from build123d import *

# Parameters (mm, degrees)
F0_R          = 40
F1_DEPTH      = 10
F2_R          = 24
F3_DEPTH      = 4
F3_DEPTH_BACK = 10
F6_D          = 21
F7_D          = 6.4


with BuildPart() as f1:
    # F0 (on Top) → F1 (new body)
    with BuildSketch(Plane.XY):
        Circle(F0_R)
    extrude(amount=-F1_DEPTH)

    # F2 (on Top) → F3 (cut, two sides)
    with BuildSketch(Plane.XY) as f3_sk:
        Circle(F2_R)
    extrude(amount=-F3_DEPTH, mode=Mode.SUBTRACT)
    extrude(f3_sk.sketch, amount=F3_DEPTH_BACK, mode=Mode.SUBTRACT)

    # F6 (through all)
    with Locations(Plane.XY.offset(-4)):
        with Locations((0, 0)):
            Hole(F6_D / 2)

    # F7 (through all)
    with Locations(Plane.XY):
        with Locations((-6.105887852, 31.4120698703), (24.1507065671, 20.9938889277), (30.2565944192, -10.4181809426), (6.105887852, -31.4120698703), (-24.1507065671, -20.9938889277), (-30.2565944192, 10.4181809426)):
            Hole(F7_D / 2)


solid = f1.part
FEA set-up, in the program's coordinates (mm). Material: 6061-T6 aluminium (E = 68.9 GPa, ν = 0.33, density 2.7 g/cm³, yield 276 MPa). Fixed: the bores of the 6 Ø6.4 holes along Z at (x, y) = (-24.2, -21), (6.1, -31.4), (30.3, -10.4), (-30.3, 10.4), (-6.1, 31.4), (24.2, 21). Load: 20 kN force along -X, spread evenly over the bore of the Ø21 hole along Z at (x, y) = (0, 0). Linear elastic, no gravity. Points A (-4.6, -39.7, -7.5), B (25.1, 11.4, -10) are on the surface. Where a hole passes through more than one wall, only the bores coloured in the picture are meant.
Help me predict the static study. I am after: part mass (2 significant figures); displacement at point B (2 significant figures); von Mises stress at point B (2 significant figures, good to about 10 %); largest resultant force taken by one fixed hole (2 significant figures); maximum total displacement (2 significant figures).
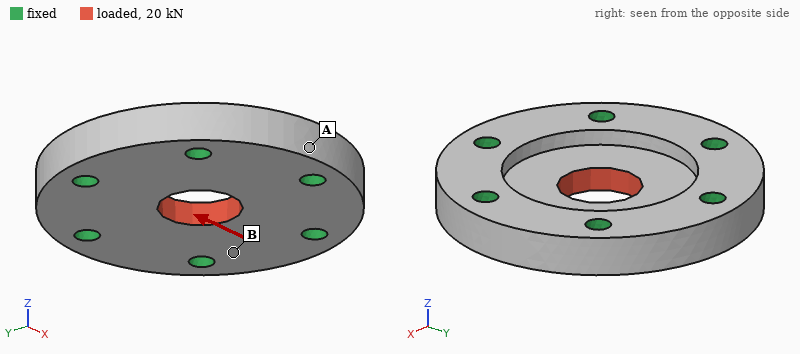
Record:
110 g
5.7 µm
23 MPa
4.8 kN
16 µm
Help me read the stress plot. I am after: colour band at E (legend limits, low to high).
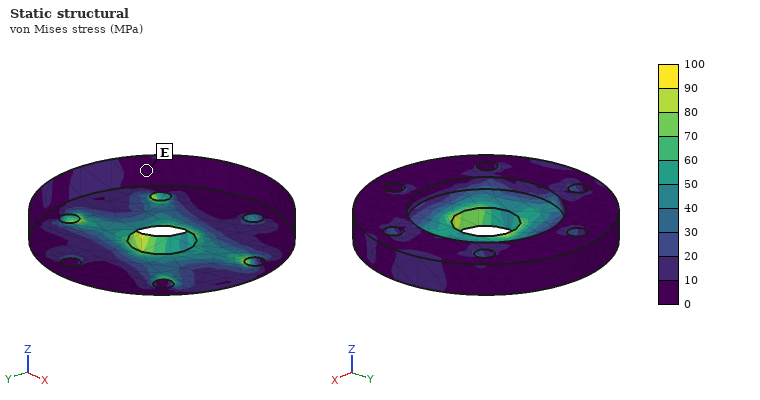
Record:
0 to 10 MPa
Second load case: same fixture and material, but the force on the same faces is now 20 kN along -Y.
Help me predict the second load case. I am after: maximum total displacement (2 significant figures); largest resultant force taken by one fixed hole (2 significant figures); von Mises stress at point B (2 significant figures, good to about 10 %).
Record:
16 µm
5.0 kN
12 MPa
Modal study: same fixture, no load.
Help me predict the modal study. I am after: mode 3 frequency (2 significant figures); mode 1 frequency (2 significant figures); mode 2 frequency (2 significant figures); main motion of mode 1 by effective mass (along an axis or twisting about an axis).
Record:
27 kHz
20 kHz
27 kHz
along Z
